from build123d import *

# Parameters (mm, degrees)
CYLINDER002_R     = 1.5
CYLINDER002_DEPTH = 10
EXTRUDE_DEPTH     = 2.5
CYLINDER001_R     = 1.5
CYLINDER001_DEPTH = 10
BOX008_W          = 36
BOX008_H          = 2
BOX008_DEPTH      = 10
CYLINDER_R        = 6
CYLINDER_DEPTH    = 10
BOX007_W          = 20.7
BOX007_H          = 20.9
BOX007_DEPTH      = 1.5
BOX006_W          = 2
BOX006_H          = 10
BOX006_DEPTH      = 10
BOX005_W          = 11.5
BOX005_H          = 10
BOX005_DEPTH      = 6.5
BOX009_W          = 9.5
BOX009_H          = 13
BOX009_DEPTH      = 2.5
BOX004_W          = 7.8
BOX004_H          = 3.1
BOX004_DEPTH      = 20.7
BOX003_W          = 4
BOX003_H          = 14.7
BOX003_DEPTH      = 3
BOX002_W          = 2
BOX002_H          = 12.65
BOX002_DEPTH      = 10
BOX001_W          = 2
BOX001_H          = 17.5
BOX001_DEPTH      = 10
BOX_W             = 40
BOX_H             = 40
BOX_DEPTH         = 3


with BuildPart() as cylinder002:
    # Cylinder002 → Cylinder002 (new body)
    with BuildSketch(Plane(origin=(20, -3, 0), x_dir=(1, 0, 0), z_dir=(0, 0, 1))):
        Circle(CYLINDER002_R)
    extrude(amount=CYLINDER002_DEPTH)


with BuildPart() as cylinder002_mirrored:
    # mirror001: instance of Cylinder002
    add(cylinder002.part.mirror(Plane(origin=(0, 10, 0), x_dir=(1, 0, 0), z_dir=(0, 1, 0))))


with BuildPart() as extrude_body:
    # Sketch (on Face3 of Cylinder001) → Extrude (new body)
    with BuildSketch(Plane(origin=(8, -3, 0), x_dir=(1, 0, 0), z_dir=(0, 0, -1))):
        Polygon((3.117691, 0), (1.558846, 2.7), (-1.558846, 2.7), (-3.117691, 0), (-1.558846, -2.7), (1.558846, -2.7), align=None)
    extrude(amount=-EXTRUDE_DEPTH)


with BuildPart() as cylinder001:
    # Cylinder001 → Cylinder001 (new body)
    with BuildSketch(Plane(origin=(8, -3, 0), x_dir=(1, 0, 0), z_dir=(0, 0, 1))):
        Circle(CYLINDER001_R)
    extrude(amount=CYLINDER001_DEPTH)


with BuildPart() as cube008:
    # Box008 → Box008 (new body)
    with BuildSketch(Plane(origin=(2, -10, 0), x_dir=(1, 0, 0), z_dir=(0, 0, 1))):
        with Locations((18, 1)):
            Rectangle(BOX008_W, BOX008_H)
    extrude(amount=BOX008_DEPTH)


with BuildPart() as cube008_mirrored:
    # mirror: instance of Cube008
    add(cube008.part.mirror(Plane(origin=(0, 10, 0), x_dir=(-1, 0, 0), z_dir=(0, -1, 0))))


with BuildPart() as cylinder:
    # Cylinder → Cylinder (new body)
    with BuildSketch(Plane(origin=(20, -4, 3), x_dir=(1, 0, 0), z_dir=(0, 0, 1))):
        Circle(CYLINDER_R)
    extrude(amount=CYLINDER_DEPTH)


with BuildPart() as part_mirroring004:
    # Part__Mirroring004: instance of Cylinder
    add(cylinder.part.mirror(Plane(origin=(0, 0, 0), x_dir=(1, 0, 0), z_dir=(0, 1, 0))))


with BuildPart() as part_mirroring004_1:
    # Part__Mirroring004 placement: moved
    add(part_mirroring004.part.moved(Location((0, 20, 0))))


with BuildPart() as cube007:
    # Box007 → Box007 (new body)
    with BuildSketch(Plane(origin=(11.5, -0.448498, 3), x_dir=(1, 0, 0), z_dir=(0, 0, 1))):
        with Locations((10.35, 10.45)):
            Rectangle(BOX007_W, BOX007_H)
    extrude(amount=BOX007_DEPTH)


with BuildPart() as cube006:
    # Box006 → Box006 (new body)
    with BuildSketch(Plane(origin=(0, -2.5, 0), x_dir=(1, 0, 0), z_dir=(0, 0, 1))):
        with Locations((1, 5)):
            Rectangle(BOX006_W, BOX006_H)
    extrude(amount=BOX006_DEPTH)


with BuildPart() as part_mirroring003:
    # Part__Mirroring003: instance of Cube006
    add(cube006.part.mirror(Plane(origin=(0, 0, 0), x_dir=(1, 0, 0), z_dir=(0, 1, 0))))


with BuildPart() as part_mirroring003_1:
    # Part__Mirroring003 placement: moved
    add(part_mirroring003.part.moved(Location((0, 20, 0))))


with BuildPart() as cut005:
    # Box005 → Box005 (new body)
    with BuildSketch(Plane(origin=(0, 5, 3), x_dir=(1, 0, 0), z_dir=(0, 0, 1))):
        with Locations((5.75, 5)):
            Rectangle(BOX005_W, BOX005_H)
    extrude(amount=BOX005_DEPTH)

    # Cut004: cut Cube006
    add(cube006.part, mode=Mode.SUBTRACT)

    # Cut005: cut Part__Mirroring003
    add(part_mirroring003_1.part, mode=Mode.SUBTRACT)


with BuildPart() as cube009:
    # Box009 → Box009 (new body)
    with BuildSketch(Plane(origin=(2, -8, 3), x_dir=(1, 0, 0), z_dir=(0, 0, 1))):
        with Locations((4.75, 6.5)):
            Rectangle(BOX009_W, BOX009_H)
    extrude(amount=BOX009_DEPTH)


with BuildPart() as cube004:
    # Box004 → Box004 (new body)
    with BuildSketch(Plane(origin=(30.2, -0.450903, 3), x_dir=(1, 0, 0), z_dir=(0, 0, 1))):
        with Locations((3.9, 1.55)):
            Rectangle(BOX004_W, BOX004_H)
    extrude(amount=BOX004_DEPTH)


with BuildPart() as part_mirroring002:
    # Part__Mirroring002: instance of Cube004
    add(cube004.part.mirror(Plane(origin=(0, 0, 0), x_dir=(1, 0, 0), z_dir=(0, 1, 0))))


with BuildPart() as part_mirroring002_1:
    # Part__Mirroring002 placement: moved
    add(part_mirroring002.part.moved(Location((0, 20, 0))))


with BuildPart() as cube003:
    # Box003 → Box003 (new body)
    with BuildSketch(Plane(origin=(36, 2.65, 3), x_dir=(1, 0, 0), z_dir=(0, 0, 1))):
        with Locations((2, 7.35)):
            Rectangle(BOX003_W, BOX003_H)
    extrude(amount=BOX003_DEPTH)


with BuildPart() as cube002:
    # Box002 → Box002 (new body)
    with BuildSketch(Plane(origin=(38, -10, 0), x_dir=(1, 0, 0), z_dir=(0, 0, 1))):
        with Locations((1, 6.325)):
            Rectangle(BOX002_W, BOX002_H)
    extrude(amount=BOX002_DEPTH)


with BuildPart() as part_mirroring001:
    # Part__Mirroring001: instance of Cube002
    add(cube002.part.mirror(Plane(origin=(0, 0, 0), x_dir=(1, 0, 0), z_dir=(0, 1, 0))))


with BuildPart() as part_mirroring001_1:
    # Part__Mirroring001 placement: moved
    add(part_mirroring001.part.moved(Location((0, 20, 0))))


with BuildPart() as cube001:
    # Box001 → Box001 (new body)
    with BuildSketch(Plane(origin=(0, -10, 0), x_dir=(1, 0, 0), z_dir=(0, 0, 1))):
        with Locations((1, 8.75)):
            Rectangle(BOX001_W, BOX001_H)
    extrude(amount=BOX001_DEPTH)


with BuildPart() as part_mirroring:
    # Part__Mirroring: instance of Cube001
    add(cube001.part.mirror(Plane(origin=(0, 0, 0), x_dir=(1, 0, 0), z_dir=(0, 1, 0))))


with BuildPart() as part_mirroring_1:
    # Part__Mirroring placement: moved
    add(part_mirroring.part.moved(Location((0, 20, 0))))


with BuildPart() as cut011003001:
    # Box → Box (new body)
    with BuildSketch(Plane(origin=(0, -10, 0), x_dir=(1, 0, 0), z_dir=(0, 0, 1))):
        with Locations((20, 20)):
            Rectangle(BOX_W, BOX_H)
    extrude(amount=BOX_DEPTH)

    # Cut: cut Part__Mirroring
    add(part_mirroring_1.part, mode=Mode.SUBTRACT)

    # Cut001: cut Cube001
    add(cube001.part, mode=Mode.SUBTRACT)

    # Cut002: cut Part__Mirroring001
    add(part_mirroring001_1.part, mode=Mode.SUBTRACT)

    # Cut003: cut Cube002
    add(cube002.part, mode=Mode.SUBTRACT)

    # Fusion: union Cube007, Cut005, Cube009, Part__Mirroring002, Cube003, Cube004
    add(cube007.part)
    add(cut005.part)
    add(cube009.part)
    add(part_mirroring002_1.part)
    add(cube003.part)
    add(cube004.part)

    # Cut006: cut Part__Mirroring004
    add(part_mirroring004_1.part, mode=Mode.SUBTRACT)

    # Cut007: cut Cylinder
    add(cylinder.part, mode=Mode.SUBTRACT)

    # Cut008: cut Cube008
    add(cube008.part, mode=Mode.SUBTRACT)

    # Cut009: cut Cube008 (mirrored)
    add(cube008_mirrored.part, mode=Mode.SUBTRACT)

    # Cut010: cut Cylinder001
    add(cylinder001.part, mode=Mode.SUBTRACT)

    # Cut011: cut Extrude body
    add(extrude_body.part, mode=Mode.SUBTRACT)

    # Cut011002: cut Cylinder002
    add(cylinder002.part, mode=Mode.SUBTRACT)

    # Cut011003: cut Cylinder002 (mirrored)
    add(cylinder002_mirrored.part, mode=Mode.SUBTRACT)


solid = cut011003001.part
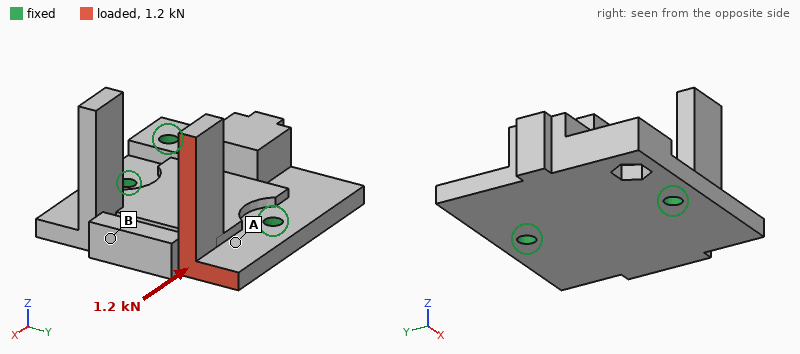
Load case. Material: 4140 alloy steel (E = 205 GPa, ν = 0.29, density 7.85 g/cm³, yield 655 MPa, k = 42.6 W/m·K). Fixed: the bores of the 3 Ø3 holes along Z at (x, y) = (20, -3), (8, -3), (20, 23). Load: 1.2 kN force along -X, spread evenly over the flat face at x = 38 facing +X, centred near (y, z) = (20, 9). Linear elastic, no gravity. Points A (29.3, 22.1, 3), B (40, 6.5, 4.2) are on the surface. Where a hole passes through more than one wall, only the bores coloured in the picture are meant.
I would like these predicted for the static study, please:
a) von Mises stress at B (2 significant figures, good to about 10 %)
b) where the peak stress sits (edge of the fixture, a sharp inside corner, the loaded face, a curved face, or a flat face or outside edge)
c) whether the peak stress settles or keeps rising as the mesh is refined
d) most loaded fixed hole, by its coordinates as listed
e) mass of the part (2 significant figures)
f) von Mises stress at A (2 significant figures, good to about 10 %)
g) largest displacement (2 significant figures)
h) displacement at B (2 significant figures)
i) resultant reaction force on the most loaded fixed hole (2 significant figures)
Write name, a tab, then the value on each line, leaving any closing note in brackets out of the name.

von Mises stress at B	38 MPa
where the peak stress sits	a sharp inside corner
whether the peak stress settles or keeps rising as the mesh is refined	keeps rising
most loaded fixed hole, by its coordinates as listed	(20, 23)
mass of the part	52 g
von Mises stress at A	120 MPa
largest displacement	0.18 mm
displacement at B	0.054 mm
resultant reaction force on the most loaded fixed hole	1.0 kN
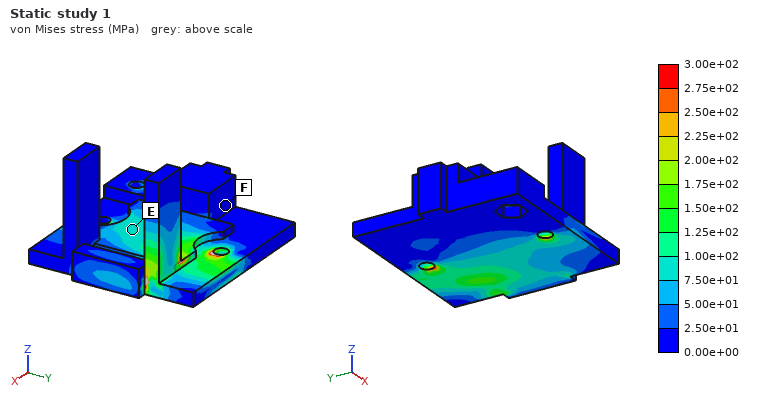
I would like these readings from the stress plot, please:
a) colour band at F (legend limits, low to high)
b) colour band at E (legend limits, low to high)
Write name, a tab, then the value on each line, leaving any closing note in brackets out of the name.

colour band at F	0.00e+00 to 2.50e+01 MPa
colour band at E	7.50e+01 to 1.00e+02 MPa
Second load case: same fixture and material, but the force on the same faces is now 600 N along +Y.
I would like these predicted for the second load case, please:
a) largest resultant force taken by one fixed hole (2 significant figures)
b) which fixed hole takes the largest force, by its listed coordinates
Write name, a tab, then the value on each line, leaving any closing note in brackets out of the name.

largest resultant force taken by one fixed hole	570 N
which fixed hole takes the largest force, by its listed coordinates	(20, -3)
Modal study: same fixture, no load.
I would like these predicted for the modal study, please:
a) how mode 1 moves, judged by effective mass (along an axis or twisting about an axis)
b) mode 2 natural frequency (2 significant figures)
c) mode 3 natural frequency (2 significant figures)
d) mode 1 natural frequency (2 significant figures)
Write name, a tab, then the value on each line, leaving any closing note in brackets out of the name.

how mode 1 moves, judged by effective mass	along Z
mode 2 natural frequency	4900 Hz
mode 3 natural frequency	5100 Hz
mode 1 natural frequency	4100 Hz
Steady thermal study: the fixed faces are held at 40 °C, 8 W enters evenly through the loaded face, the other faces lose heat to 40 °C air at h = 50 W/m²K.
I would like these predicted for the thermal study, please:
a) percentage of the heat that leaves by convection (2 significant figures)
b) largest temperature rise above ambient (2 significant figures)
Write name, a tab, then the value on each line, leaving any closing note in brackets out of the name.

percentage of the heat that leaves by convection	31 %
largest temperature rise above ambient	73 K
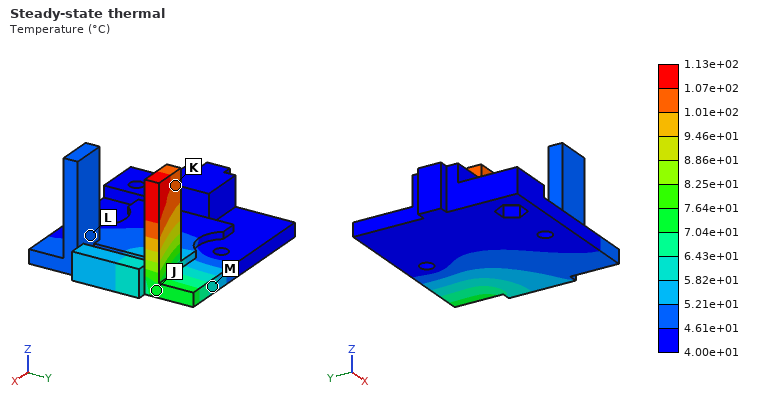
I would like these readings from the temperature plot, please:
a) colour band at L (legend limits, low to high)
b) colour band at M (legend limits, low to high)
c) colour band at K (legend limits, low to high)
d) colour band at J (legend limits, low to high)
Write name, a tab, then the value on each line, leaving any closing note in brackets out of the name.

colour band at L	4.61e+01 to 5.21e+01 °C
colour band at M	5.82e+01 to 6.43e+01 °C
colour band at K	1.01e+02 to 1.07e+02 °C
colour band at J	7.04e+01 to 7.64e+01 °C
